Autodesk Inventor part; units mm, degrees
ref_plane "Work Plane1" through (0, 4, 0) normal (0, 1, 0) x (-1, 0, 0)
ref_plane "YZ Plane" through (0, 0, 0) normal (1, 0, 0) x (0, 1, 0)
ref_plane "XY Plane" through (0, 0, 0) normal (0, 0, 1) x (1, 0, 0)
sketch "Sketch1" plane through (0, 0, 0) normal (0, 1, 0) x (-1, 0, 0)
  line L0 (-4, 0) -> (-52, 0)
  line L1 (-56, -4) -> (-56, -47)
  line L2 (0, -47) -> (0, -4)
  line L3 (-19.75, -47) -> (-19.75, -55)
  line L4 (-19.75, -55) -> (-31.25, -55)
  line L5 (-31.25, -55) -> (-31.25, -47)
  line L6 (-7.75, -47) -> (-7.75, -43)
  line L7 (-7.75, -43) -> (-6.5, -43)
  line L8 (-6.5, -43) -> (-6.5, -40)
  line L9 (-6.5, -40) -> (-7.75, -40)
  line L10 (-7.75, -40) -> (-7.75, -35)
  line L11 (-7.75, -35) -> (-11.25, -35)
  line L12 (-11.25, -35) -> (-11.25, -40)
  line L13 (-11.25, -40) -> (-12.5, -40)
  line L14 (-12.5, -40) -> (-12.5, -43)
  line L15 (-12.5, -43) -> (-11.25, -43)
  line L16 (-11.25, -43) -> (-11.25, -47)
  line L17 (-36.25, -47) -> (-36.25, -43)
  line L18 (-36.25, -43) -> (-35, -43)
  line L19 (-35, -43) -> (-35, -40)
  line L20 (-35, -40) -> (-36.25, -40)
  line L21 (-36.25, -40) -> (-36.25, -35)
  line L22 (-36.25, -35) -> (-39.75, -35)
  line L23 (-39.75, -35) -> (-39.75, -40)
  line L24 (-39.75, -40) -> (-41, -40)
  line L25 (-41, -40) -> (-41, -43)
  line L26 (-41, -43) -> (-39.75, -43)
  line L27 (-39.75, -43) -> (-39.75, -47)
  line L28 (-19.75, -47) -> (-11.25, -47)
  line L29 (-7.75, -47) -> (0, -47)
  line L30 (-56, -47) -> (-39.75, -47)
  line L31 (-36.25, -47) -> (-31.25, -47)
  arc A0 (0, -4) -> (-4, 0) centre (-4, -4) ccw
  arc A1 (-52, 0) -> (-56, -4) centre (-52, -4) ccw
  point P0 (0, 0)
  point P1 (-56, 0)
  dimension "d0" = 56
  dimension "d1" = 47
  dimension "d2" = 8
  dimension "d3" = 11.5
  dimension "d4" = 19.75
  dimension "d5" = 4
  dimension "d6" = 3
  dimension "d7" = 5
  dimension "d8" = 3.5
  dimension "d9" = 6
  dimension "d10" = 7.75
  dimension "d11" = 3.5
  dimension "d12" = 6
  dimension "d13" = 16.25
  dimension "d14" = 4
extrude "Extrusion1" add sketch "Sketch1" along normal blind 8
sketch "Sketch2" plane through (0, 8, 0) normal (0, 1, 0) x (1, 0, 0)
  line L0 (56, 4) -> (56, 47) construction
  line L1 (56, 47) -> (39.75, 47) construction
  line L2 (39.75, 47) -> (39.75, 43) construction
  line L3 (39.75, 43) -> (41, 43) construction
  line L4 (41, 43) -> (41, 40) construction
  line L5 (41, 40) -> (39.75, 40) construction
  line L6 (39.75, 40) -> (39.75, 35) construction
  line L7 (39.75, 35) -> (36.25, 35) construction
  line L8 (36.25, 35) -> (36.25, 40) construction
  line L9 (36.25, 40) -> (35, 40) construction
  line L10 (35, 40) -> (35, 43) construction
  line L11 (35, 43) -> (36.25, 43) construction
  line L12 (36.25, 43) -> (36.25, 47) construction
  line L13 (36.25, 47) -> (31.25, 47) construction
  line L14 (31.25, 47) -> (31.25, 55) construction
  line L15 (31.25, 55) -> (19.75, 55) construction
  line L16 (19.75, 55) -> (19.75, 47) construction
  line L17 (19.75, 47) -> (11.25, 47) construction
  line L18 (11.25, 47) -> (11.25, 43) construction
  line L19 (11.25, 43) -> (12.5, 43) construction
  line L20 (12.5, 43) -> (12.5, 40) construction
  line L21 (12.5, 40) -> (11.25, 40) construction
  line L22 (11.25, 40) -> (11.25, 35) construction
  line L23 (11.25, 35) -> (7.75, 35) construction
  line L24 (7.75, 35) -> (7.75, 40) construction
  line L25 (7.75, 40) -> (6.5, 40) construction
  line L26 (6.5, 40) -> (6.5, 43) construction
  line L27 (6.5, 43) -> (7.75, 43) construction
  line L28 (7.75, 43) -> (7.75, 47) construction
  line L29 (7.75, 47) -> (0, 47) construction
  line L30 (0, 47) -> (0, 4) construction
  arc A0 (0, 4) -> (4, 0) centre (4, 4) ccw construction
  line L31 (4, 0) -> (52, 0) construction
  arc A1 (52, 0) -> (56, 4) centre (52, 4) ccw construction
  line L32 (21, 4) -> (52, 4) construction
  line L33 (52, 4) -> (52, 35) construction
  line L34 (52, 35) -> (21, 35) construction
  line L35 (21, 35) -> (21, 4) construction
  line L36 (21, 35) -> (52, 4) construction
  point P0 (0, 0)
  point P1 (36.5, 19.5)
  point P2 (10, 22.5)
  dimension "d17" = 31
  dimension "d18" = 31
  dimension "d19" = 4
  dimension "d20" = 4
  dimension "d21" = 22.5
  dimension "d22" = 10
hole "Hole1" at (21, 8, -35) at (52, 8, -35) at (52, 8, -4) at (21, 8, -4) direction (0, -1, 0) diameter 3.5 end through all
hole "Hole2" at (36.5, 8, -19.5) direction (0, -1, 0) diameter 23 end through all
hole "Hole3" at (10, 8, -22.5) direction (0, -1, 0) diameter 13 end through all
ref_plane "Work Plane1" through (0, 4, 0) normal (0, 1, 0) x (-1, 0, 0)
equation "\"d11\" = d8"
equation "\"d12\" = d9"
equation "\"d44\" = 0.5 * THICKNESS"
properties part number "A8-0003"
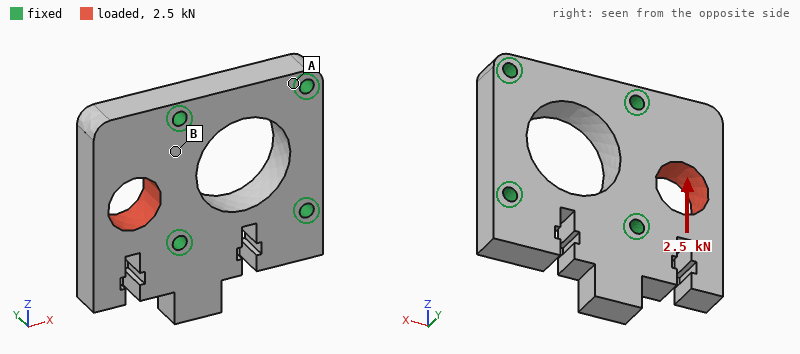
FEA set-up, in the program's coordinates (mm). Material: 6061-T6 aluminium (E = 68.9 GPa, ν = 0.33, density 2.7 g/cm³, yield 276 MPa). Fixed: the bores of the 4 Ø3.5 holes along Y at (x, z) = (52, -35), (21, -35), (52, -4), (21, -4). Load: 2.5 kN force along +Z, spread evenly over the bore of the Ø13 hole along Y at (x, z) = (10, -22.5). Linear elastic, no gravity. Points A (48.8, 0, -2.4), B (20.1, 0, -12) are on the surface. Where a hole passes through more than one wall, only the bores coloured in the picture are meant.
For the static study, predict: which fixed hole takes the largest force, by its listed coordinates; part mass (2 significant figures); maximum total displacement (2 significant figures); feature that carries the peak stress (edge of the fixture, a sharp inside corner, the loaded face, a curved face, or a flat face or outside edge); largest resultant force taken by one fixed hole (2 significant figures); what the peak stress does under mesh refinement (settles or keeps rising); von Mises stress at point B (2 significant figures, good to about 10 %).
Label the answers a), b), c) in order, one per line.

a) (21, -35)
b) 44 g
c) 15 µm
d) edge of the fixture
e) 1.6 kN
f) keeps rising
g) 8.6 MPa
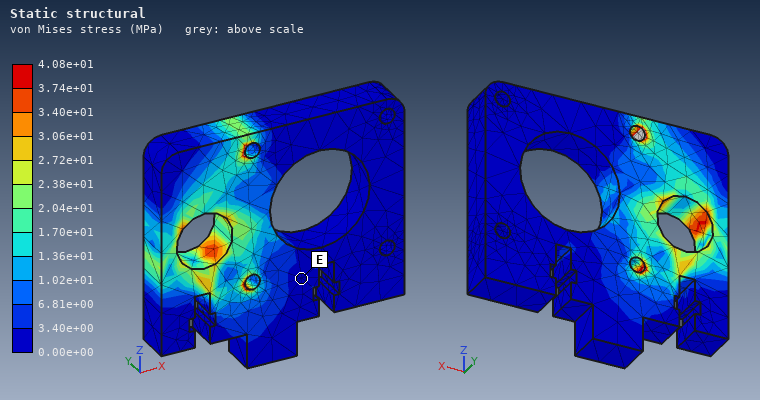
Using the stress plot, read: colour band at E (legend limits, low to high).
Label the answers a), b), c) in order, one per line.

a) 0.00e+00 to 3.40e+00 MPa
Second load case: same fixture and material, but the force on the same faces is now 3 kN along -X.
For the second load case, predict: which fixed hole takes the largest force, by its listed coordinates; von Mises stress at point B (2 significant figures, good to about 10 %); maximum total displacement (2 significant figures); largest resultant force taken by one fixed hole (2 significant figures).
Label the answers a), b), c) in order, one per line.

a) (21, -35)
b) 13 MPa
c) 9.5 µm
d) 1.7 kN
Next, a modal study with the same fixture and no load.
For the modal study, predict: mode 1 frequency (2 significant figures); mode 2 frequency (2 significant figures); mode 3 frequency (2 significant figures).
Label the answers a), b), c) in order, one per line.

a) 9200 Hz
b) 13 kHz
c) 15 kHz
